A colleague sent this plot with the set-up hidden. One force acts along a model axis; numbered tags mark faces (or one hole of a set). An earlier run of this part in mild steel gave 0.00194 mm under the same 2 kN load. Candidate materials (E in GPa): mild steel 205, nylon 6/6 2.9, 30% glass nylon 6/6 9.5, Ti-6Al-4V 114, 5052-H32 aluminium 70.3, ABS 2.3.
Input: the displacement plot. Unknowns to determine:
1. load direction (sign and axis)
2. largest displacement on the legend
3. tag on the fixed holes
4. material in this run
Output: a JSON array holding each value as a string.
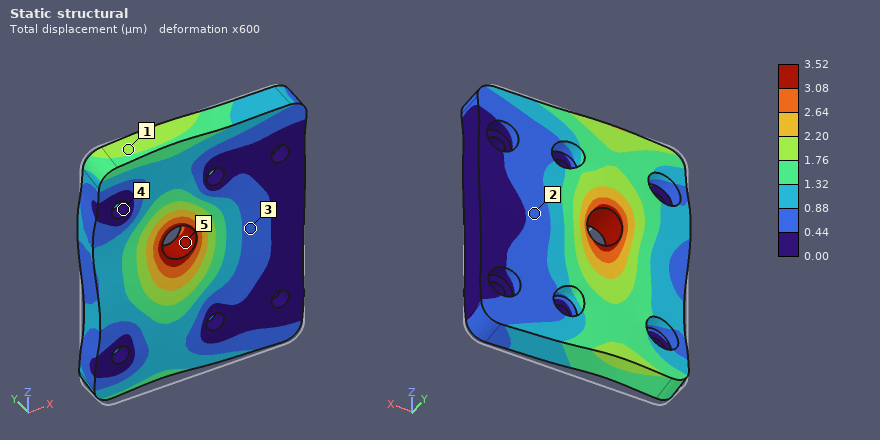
["+Z", "3.52 µm", "4", "Ti-6Al-4V"]
